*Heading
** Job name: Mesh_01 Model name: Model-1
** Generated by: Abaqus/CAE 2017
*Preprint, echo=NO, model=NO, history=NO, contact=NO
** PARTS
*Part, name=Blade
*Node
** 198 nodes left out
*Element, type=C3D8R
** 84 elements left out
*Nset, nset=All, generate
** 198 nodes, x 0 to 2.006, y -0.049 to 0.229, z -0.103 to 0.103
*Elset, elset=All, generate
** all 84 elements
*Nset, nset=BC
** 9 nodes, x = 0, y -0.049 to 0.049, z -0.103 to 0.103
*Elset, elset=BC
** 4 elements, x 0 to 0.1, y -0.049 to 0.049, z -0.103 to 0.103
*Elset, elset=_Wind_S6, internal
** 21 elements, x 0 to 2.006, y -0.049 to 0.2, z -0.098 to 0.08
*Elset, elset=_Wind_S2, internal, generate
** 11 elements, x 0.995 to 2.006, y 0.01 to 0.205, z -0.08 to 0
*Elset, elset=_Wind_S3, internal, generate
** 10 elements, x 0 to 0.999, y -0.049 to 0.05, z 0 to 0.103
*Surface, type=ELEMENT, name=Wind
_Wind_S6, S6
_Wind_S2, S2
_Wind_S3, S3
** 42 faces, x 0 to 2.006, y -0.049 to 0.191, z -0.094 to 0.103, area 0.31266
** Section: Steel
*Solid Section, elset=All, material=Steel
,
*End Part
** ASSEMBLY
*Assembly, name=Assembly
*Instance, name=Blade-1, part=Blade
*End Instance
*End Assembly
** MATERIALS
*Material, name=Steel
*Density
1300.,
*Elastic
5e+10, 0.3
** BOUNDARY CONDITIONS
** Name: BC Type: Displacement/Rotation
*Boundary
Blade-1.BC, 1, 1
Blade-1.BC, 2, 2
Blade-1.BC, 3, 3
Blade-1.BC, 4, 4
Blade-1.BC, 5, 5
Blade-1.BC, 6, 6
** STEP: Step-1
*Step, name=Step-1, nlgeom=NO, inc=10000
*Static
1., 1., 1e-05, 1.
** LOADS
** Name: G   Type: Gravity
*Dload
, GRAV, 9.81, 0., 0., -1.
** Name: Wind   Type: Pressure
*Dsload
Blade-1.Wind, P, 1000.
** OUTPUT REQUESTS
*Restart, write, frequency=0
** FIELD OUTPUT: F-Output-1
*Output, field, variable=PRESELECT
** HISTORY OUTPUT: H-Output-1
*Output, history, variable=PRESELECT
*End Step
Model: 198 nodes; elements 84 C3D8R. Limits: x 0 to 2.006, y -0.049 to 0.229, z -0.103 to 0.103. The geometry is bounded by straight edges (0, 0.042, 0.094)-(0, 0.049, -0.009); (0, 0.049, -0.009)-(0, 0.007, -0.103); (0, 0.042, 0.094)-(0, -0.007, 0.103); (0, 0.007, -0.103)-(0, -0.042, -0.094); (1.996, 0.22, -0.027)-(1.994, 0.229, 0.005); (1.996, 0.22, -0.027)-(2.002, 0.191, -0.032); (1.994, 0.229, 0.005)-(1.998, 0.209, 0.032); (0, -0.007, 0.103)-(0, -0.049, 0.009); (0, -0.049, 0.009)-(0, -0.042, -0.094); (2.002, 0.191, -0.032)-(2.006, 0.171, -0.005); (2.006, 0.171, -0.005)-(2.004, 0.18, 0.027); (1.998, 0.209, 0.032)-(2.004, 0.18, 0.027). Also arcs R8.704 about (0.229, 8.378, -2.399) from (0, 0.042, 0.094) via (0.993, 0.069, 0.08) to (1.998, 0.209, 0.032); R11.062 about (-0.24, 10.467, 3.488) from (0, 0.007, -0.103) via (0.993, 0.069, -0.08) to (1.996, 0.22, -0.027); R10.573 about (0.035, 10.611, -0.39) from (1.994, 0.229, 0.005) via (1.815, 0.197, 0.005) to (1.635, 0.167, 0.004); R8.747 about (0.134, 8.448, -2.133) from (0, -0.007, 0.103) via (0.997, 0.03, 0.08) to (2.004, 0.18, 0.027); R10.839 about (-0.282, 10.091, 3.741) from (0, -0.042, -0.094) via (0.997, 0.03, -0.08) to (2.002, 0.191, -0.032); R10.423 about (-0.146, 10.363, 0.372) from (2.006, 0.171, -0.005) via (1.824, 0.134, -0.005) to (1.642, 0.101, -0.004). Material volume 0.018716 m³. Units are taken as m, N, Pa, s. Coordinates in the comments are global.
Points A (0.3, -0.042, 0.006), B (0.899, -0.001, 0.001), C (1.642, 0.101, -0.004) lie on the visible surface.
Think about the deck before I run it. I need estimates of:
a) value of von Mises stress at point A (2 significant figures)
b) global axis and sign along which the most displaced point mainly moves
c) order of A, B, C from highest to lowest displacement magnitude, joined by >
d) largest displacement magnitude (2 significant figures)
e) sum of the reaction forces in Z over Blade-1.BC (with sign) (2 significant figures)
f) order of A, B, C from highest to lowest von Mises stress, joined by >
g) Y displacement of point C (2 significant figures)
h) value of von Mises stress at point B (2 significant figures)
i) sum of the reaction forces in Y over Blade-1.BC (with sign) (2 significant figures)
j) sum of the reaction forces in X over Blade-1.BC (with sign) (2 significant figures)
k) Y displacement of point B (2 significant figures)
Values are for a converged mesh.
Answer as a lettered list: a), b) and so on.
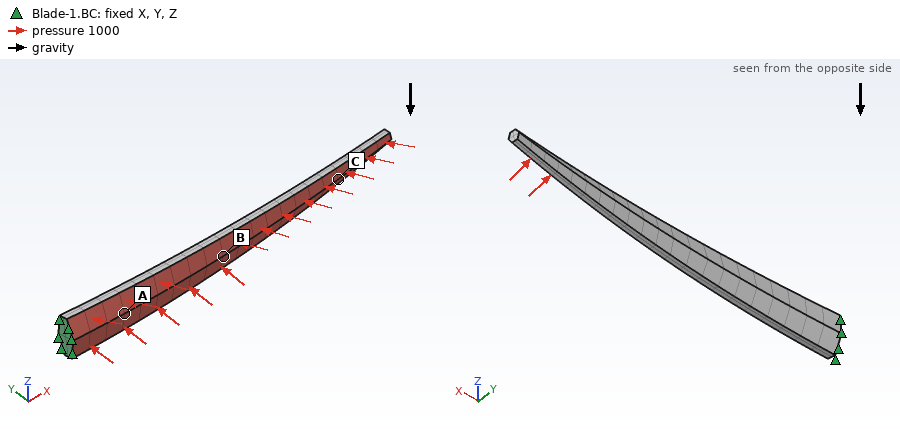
a) 1.4e+06 Pa
b) +Y
c) C > B > A
d) 9.1e-04 m
e) 250 N
f) A > B > C
g) 6.6e-04 m
h) 7.2e+05 Pa
i) -300 N
j) 29 N
k) 2.3e-04 m
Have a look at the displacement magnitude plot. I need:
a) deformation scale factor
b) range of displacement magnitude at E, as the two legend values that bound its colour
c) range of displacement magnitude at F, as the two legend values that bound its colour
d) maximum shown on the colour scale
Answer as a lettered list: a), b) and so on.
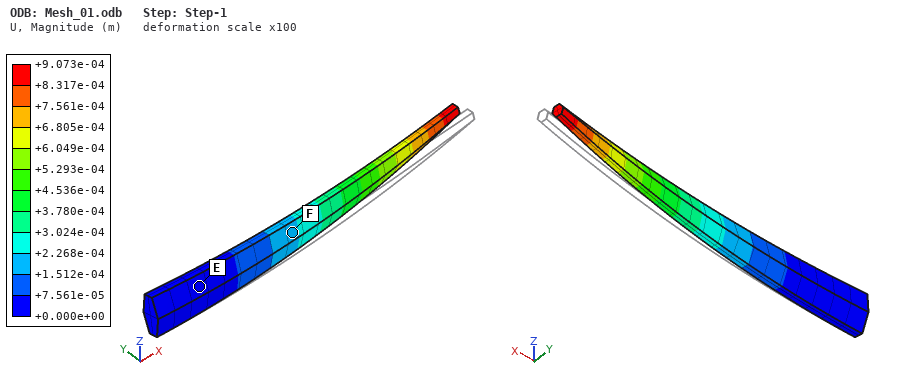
a) 100
b) +0.000e+00 to +7.561e-05 m
c) +1.512e-04 to +2.268e-04 m
d) +9.073e-04 m
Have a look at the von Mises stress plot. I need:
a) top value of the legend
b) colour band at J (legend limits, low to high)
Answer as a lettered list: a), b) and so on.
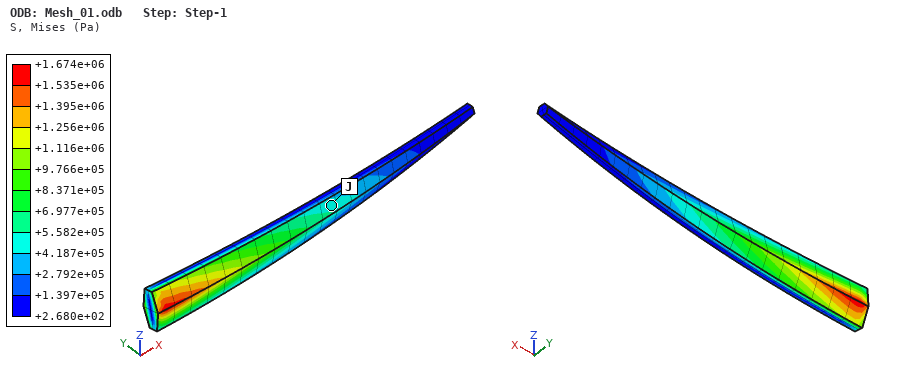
a) +1.674e+06 Pa
b) +4.187e+05 to +5.582e+05 Pa
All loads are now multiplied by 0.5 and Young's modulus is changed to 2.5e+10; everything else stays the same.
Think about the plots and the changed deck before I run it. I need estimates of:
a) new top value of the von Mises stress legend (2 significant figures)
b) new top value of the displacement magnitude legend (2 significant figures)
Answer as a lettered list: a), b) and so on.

a) 8.4e+05 Pa
b) 9.1e-04 m
